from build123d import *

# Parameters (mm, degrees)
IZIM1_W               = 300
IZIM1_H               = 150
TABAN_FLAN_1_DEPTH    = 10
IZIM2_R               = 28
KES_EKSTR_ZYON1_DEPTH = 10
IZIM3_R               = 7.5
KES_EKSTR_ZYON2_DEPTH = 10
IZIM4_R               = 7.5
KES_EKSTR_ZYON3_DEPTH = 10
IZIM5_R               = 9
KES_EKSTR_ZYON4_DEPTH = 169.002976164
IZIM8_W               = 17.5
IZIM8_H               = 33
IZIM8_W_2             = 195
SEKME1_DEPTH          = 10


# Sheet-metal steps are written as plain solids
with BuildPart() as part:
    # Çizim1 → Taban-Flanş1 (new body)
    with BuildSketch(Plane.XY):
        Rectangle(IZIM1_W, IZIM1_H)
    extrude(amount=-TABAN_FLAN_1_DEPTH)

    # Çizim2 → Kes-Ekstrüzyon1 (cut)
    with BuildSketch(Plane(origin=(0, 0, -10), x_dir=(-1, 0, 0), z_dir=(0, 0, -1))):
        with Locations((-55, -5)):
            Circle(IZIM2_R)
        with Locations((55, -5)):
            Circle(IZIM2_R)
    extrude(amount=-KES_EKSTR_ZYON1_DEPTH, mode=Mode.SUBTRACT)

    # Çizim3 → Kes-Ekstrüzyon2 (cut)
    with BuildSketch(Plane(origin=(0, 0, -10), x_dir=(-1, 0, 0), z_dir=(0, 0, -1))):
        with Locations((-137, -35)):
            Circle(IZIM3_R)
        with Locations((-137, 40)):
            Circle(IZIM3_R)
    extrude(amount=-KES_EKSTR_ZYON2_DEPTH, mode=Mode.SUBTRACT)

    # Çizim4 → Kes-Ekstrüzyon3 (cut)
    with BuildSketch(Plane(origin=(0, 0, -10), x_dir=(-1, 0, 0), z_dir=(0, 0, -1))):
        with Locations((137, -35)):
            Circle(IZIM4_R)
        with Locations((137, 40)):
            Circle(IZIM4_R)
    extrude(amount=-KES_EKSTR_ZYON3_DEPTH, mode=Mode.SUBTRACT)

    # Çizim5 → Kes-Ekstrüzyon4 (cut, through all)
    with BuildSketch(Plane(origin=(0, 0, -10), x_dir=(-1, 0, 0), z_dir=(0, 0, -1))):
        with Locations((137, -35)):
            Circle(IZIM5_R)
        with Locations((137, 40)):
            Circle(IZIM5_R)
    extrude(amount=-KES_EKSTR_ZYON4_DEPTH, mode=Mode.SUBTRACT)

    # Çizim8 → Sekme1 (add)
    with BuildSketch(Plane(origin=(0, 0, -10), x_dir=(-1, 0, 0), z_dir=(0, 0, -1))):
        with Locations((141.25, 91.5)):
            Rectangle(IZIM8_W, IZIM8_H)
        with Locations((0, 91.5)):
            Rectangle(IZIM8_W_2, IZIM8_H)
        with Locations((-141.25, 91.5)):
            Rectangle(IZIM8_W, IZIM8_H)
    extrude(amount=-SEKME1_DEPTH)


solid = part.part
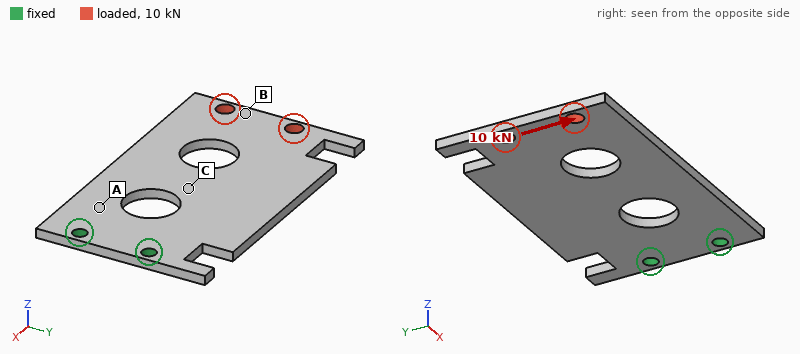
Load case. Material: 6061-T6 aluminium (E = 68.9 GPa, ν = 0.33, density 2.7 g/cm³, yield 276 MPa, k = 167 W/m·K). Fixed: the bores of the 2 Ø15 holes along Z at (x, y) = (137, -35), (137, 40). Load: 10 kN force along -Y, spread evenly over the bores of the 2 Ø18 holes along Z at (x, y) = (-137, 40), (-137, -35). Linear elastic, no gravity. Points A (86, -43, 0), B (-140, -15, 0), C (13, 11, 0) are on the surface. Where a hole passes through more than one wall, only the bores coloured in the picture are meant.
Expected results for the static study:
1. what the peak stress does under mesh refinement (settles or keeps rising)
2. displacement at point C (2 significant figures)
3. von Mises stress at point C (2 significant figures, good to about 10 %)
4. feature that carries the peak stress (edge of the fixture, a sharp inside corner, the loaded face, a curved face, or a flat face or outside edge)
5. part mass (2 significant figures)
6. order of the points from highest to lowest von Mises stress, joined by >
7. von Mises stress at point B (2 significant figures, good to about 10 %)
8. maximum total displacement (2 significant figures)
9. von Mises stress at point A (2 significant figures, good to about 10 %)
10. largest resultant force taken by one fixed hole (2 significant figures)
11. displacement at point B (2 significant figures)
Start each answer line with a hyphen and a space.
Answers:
- keeps rising
- 0.27 mm
- 27 MPa
- edge of the fixture
- 1.3 kg
- A > C > B
- 14 MPa
- 0.75 mm
- 48 MPa
- 32 kN
- 0.68 mm
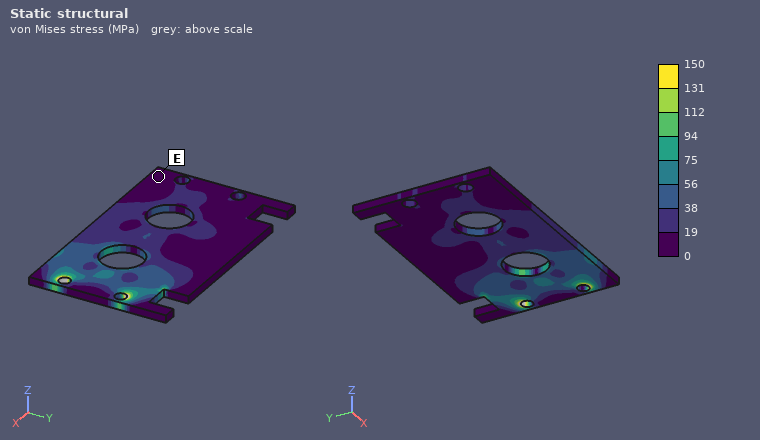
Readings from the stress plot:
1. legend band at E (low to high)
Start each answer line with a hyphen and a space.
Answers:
- 0 to 19 MPa
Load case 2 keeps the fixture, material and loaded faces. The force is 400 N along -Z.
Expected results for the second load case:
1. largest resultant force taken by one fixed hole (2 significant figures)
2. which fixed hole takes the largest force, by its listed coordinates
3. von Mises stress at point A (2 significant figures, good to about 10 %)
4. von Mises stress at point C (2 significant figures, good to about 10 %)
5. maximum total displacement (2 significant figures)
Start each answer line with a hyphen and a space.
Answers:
- 220 N
- (137, 40)
- 37 MPa
- 14 MPa
- 3.7 mm
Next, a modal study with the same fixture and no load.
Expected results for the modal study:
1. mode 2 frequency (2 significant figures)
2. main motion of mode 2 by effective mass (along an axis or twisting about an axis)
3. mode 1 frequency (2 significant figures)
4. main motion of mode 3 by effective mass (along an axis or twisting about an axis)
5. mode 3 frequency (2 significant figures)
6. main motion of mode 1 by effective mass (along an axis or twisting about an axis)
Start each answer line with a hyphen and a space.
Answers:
- 310 Hz
- twisting about X
- 95 Hz
- along Z
- 590 Hz
- along Z
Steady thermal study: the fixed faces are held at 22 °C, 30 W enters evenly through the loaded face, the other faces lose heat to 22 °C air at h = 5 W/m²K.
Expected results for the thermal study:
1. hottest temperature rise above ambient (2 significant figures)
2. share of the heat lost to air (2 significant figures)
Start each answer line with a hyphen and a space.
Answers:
- 33 K
- 26 %
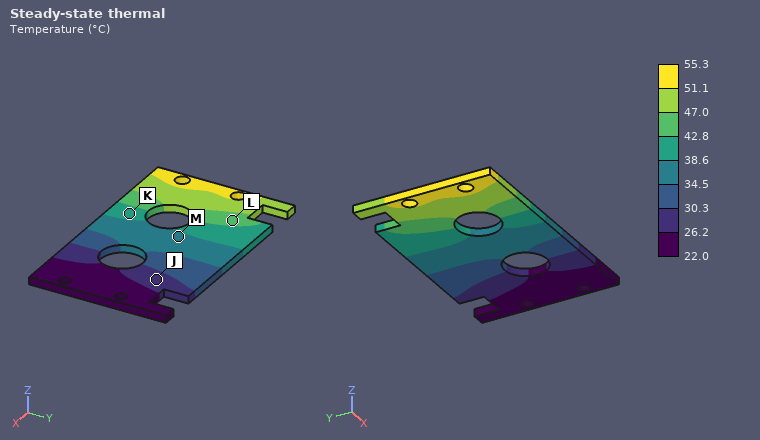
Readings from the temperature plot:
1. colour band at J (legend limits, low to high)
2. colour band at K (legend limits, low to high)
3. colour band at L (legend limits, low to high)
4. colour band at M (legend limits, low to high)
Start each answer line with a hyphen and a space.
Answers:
- 26.2 to 30.3 °C
- 38.6 to 42.8 °C
- 42.8 to 47.0 °C
- 34.5 to 38.6 °C
